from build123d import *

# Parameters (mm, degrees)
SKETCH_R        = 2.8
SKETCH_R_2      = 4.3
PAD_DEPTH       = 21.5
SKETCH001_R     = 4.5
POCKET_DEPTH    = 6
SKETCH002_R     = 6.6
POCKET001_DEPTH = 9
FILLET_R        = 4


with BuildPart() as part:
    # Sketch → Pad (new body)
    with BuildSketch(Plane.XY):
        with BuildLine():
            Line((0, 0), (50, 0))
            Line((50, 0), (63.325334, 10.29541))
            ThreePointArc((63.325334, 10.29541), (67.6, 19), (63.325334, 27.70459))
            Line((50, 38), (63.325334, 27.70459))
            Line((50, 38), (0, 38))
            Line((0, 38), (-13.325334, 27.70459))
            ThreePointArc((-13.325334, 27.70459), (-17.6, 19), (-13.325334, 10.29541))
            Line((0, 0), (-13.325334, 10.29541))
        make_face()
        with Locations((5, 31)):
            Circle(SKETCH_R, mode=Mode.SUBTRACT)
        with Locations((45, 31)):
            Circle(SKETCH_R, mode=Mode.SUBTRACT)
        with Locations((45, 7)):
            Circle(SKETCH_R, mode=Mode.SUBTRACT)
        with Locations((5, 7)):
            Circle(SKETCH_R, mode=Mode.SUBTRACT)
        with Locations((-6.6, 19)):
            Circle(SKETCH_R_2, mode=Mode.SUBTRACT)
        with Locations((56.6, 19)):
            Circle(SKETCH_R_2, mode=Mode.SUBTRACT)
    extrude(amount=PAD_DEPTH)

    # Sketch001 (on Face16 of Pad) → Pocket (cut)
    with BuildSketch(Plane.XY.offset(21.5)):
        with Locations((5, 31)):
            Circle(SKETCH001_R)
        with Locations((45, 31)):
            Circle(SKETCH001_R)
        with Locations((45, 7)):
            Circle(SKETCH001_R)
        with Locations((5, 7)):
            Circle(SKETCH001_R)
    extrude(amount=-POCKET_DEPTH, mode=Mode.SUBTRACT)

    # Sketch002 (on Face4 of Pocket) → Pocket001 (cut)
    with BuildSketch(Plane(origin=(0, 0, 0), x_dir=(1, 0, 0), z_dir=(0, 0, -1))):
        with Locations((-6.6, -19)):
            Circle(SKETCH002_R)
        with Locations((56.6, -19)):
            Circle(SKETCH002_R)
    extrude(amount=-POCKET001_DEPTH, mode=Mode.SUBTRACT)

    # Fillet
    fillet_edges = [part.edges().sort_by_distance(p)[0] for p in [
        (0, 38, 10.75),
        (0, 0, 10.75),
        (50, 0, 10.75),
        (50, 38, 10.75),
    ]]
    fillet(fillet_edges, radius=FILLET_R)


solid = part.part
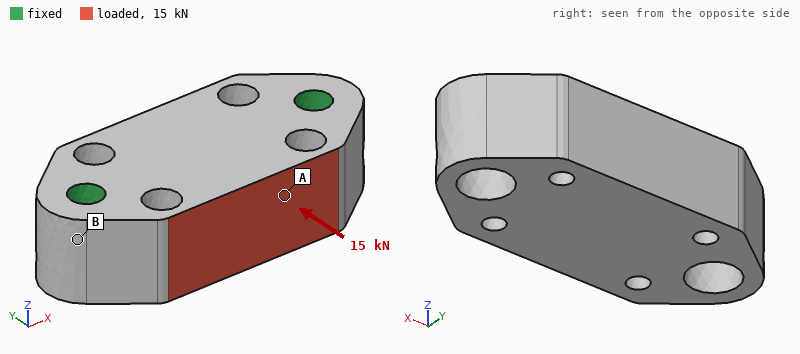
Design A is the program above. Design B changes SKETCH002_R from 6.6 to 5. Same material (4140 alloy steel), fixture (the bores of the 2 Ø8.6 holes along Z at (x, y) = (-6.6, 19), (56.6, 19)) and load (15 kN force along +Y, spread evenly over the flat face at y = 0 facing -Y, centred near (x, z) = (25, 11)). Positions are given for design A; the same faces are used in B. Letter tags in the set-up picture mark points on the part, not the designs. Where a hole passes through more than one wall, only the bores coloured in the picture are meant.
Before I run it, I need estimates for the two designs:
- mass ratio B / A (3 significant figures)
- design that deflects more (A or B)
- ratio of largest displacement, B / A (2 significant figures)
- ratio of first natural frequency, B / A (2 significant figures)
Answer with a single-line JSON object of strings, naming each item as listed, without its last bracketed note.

{"mass ratio B / A": "1.02", "design that deflects more": "A", "ratio of largest displacement, B / A": "0.91", "ratio of first natural frequency, B / A": "1.1"}
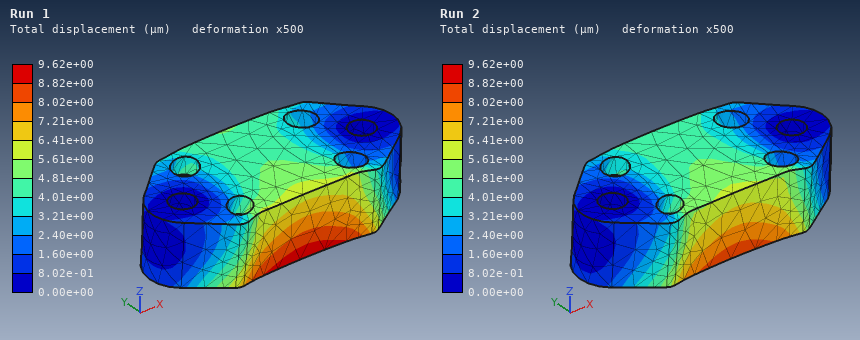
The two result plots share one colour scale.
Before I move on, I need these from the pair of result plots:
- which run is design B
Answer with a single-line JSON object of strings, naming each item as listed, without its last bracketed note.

{"which run is design B": "Run 2"}
